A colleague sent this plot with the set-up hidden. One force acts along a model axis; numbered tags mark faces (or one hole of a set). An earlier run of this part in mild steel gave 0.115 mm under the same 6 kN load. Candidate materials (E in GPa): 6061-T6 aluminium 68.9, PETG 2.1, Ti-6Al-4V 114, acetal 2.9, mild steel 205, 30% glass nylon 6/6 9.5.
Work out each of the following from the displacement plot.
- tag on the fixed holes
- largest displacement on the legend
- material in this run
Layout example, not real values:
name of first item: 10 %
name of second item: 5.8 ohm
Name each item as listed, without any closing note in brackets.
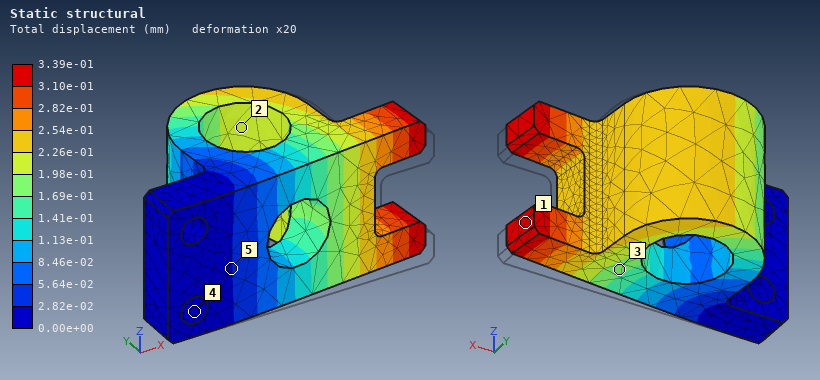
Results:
tag on the fixed holes: 4
largest displacement on the legend: 3.39e-01 mm
material in this run: 6061-T6 aluminium
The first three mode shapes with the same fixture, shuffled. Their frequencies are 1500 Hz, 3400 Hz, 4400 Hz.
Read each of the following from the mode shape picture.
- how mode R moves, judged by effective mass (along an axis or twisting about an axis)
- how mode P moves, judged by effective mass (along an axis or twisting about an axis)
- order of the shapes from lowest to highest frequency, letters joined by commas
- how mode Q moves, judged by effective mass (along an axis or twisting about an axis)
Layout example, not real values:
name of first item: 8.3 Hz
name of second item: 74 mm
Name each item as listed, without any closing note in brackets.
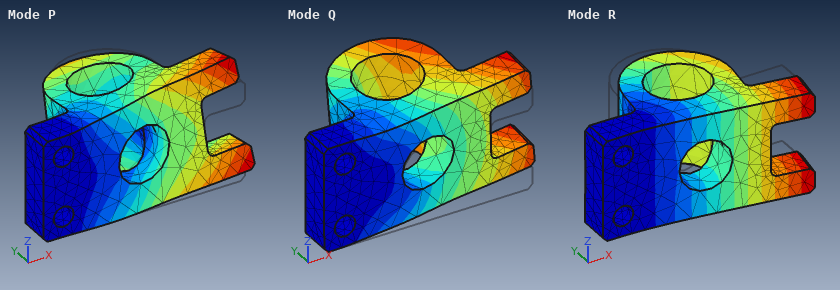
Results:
how mode R moves, judged by effective mass: along Y
how mode P moves, judged by effective mass: twisting about X
order of the shapes from lowest to highest frequency, letters joined by commas: R, Q, P
how mode Q moves, judged by effective mass: along Z
